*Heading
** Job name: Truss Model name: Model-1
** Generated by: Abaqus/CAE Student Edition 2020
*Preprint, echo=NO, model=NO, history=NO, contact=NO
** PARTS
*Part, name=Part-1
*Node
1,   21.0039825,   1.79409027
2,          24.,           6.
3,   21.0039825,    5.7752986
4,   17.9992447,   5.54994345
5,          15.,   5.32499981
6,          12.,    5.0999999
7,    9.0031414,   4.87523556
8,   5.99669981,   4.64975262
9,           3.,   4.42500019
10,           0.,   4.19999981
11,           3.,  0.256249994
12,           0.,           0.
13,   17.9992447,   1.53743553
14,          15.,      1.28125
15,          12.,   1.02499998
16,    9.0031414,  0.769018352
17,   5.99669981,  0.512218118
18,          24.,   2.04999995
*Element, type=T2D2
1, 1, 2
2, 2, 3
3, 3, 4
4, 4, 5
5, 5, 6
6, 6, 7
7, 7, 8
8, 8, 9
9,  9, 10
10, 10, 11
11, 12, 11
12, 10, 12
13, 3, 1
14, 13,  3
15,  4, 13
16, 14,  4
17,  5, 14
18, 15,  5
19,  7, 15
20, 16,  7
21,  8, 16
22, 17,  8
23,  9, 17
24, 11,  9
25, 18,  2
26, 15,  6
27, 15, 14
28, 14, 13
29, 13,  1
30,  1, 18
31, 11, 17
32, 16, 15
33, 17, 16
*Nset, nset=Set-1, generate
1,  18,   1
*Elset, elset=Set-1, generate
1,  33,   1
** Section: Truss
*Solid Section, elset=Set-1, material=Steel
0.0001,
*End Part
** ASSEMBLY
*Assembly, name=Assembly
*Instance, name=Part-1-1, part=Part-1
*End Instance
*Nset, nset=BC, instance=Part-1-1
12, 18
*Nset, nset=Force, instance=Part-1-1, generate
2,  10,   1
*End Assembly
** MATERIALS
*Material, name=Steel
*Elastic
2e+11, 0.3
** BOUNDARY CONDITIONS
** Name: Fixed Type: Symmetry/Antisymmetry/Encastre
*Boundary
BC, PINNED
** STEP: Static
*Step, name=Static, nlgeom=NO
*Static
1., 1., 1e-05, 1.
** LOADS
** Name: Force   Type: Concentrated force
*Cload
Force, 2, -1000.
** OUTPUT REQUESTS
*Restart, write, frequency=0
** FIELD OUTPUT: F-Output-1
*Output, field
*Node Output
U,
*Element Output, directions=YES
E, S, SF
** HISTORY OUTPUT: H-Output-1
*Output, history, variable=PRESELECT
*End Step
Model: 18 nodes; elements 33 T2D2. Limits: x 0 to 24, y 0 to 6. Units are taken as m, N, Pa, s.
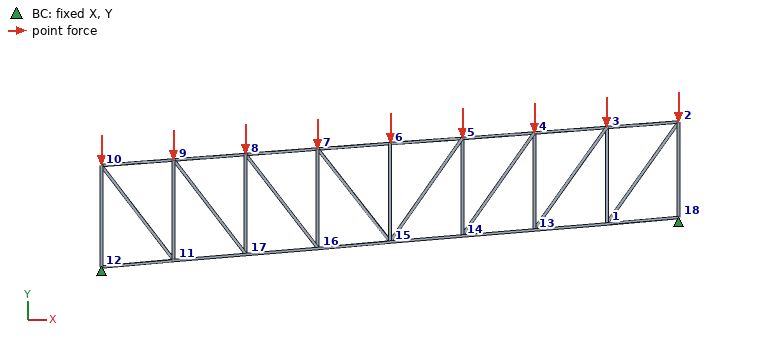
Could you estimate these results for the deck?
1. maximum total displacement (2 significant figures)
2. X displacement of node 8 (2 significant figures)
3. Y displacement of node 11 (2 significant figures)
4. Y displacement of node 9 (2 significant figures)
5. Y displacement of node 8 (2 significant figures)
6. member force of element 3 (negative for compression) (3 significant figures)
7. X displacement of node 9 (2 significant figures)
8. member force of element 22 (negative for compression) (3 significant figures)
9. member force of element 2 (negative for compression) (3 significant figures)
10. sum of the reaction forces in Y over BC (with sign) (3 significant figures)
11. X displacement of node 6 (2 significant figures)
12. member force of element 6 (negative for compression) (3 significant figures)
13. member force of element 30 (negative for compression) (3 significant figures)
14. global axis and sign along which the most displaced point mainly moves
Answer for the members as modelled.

0.013 m
0.0026 m
-0.0046 m
-0.0053 m
-0.0090 m
-4500 N
0.0030 m
-2550 N
-2640 N
9000 N
0.0011 m
-5910 N
-3140 N
-Y
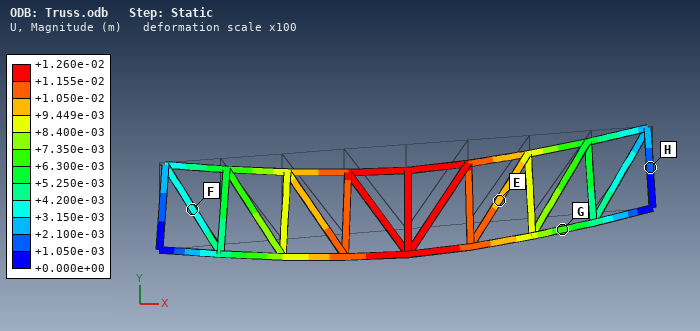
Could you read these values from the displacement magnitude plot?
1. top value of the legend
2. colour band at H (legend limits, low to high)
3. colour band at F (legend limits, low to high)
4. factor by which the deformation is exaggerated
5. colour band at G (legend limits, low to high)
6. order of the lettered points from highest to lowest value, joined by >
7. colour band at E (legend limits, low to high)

+1.260e-02 m
+1.050e-03 to +2.100e-03 m
+3.150e-03 to +4.200e-03 m
100
+6.300e-03 to +7.350e-03 m
E > G > F > H
+9.449e-03 to +1.050e-02 m
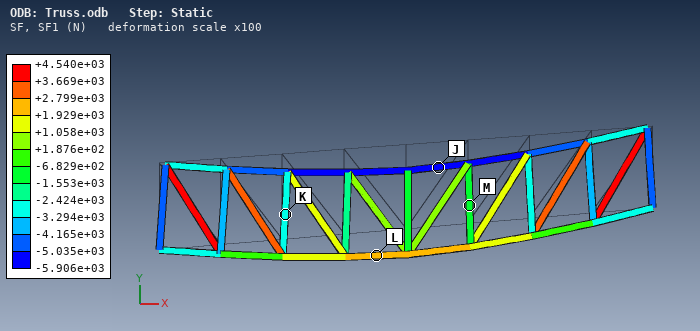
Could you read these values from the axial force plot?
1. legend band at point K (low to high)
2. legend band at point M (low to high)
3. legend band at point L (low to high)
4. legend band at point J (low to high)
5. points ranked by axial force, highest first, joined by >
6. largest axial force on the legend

-3.294e+03 to -2.424e+03 N
-1.553e+03 to -6.829e+02 N
+1.929e+03 to +2.799e+03 N
-5.906e+03 to -5.035e+03 N
L > M > K > J
+4.540e+03 N
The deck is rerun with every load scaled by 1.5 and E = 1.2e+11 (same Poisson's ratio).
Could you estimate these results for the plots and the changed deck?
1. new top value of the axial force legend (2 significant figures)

6800 N
